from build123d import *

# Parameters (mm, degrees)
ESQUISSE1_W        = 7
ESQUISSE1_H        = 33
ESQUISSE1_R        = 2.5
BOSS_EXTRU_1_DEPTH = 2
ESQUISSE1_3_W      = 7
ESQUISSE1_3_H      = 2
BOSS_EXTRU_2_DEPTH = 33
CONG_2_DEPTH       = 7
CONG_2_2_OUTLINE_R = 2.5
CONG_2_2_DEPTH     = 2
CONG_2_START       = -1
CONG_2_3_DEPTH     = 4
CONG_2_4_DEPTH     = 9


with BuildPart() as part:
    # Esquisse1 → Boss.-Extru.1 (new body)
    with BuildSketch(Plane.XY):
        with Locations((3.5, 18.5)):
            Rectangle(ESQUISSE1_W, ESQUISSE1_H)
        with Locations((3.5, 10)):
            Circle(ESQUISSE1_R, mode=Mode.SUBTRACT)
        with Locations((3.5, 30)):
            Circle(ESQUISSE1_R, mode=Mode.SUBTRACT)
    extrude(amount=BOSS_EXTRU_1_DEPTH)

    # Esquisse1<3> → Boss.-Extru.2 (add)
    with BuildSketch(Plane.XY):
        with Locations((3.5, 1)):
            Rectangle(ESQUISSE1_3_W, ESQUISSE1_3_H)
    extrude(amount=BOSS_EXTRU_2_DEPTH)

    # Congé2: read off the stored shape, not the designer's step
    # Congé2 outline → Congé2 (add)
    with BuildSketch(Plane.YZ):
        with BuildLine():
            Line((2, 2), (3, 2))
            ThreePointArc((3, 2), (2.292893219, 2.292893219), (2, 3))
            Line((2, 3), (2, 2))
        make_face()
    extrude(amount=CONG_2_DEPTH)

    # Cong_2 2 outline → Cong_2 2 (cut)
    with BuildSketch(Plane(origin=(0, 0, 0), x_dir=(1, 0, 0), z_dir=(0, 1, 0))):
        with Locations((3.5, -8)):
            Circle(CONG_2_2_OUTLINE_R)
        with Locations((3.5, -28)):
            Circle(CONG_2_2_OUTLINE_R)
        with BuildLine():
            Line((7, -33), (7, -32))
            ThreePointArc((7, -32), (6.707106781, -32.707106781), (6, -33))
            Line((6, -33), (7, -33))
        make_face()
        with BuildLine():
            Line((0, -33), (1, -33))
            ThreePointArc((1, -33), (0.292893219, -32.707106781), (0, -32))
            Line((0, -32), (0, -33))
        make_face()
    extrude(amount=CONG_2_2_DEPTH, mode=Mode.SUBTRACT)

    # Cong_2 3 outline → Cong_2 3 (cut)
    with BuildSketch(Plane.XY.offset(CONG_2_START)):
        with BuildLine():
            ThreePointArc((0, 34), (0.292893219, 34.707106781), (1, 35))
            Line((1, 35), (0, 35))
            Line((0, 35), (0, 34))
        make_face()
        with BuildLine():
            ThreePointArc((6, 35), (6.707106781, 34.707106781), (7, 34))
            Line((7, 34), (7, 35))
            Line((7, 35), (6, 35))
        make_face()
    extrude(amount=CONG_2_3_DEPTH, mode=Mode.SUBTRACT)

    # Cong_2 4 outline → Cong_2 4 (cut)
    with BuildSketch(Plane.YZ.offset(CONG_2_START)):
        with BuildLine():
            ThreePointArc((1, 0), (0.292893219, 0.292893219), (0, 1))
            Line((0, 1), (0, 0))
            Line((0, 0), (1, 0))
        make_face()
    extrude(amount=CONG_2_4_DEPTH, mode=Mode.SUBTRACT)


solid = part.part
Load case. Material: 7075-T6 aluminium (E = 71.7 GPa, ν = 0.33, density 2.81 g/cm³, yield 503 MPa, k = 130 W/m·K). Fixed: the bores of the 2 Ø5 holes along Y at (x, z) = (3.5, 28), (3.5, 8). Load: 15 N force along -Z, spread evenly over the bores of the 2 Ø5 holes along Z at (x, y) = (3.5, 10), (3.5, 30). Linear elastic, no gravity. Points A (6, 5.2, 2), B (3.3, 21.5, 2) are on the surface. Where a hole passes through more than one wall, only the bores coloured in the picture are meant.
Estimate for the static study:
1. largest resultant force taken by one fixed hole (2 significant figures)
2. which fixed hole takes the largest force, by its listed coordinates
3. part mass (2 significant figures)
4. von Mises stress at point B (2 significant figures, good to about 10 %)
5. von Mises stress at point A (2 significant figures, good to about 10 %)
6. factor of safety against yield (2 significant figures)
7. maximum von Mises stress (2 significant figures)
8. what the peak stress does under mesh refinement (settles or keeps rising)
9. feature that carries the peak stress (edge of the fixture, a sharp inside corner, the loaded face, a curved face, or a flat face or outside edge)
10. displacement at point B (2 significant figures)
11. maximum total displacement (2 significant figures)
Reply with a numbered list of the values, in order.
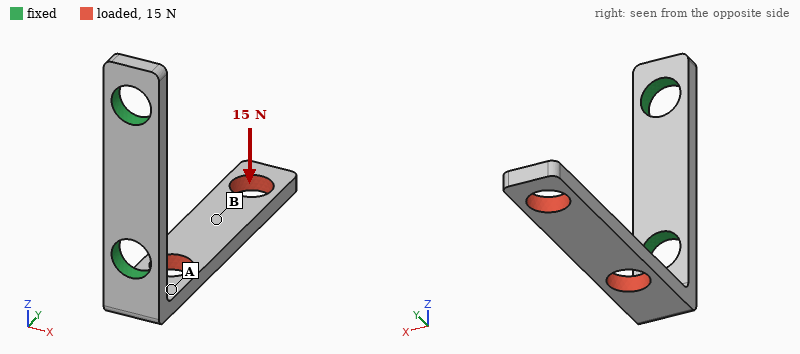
1. 15 N
2. (3.5, 8)
3. 2.2 g
4. 14 MPa
5. 50 MPa
6. 3.4
7. 150 MPa
8. settles
9. the loaded face
10. 0.24 mm
11. 0.48 mm
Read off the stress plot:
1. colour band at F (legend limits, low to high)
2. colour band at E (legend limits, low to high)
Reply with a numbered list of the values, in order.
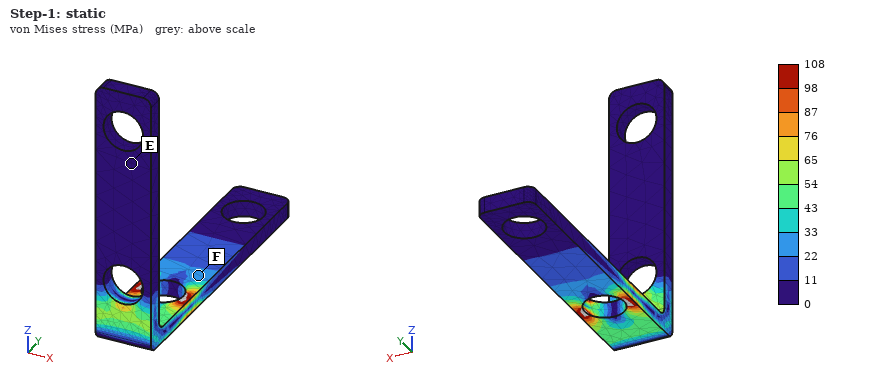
1. 22 to 33 MPa
2. 0 to 11 MPa
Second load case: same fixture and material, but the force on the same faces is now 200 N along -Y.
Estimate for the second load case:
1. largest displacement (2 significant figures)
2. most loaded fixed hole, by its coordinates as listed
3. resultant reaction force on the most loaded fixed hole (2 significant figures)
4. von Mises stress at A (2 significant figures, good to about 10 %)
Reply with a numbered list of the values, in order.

1. 0.24 mm
2. (3.5, 8)
3. 200 N
4. 19 MPa
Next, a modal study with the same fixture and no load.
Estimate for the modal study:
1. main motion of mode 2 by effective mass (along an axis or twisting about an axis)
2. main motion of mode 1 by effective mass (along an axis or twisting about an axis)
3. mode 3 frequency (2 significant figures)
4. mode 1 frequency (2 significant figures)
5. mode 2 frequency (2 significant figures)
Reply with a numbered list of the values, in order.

1. along X
2. along Z
3. 7400 Hz
4. 1200 Hz
5. 2500 Hz
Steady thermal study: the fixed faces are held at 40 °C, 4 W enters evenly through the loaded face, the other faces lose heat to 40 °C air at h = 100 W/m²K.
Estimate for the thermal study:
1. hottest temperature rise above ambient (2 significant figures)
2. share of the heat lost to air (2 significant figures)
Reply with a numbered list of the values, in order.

1. 42 K
2. 38 %
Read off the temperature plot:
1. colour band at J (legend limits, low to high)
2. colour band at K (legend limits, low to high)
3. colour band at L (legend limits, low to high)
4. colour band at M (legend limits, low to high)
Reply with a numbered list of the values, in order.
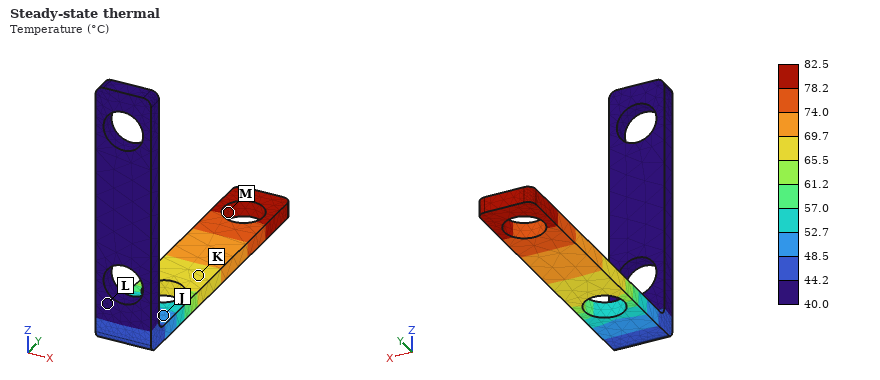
1. 48.5 to 52.7 °C
2. 65.5 to 69.7 °C
3. 40.0 to 44.2 °C
4. 78.2 to 82.5 °C
